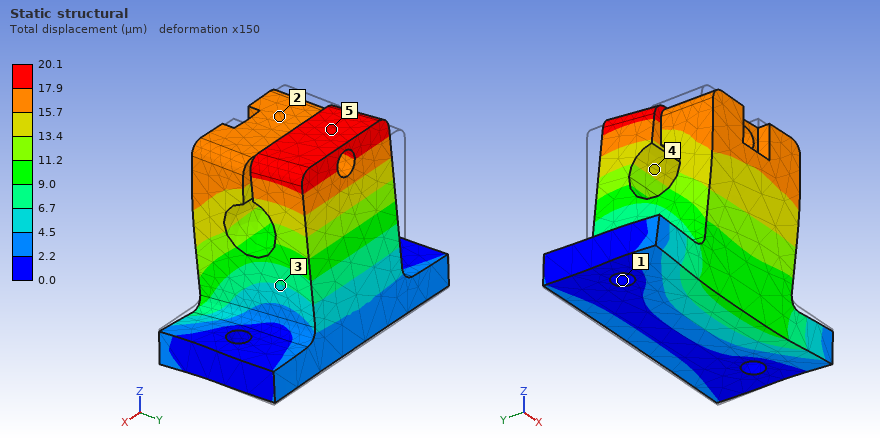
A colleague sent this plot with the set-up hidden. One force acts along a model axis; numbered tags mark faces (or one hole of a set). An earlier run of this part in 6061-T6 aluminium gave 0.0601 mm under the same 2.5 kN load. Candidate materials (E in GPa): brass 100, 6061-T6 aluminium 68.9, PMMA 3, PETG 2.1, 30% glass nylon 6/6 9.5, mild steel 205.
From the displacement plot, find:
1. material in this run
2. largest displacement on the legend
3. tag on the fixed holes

mild steel
20.1 µm
1
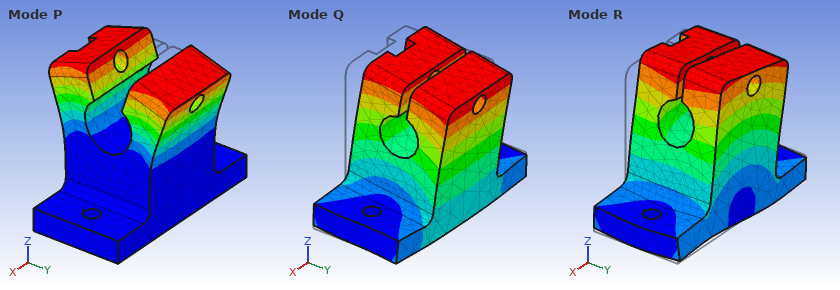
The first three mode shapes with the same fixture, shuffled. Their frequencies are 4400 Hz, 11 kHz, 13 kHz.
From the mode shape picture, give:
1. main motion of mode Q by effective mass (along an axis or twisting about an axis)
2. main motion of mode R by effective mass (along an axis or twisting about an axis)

along Y
along X
